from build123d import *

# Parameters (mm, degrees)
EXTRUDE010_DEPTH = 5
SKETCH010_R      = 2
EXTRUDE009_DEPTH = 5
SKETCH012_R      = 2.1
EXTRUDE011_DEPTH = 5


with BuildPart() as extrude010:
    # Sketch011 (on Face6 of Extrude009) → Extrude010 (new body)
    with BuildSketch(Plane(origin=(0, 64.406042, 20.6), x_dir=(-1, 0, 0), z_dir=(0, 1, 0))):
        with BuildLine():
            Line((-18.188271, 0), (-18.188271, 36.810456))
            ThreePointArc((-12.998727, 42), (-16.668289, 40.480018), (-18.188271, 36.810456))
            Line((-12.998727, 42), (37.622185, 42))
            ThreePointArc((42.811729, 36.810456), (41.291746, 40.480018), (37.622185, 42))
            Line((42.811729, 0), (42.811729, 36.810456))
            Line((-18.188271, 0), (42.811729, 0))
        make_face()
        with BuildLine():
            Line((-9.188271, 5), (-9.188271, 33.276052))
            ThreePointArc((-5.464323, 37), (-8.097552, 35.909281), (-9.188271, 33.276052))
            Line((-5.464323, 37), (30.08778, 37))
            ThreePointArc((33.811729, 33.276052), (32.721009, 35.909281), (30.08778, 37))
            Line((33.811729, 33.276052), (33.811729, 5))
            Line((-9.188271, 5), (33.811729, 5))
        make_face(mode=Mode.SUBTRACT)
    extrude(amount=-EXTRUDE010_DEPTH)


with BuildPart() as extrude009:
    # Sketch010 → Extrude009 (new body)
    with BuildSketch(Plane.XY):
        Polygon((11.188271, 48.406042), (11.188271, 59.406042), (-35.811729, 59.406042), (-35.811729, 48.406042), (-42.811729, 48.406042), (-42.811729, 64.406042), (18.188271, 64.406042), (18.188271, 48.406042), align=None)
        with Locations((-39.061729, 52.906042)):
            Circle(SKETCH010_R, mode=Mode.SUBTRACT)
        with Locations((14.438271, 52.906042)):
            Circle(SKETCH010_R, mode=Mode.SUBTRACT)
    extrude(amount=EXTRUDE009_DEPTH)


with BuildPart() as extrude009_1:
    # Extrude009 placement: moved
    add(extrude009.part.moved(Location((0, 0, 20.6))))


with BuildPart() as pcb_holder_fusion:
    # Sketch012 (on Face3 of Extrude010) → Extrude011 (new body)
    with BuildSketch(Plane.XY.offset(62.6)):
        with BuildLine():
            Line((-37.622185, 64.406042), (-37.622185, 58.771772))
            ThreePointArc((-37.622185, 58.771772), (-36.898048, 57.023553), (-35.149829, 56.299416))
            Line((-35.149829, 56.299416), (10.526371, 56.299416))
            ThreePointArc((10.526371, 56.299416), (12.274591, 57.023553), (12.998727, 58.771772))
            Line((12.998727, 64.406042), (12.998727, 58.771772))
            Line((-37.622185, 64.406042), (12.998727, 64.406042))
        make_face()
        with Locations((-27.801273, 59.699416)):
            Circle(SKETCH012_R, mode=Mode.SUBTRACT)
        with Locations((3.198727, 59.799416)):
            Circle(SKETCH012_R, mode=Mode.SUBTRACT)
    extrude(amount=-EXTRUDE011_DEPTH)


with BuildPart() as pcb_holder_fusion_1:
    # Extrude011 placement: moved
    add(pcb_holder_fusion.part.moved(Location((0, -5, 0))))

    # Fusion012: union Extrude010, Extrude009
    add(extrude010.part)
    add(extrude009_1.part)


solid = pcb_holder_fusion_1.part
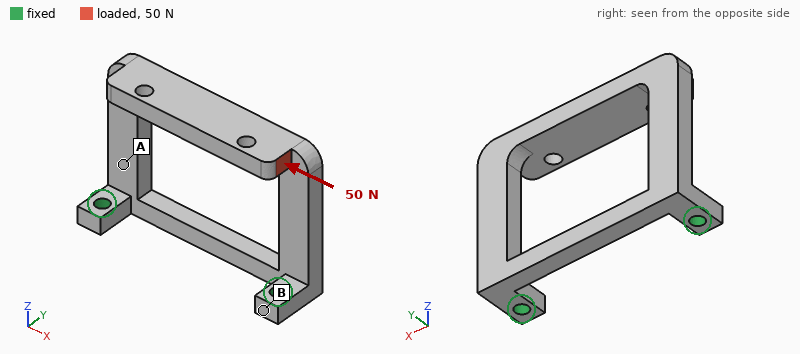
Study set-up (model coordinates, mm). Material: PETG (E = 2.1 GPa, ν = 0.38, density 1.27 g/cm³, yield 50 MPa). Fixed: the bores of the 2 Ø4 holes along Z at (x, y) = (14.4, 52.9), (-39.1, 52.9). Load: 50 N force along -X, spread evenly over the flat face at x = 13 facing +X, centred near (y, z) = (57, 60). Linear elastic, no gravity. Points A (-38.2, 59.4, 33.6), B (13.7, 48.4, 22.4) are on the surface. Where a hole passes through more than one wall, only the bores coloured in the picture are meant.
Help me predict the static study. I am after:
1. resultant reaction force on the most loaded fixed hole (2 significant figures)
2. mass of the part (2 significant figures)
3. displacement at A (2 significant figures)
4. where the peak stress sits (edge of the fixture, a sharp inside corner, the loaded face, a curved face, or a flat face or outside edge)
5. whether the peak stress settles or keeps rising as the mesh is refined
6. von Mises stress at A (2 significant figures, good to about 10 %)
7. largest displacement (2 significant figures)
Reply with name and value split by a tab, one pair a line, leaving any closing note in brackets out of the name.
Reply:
resultant reaction force on the most loaded fixed hole	35 N
mass of the part	11 g
displacement at A	0.19 mm
where the peak stress sits	edge of the fixture
whether the peak stress settles or keeps rising as the mesh is refined	keeps rising
von Mises stress at A	3.1 MPa
largest displacement	0.81 mm
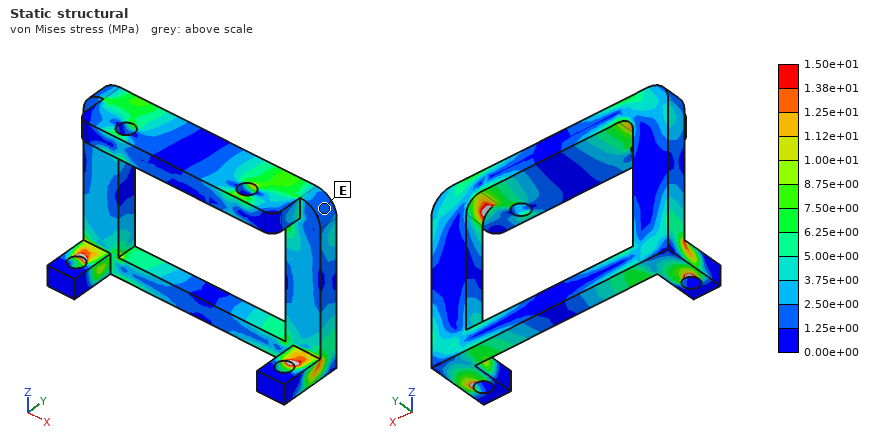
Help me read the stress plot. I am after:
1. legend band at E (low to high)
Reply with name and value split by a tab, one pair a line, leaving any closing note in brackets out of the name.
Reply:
legend band at E	1.25e+00 to 2.50e+00 MPa
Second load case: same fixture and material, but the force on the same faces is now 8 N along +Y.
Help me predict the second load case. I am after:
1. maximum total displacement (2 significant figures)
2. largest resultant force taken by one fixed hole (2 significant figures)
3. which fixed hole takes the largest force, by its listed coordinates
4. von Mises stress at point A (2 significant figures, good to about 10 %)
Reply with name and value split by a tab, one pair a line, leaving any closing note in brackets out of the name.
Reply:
maximum total displacement	0.80 mm
largest resultant force taken by one fixed hole	7.2 N
which fixed hole takes the largest force, by its listed coordinates	(14.4, 52.9)
von Mises stress at point A	2.2 MPa
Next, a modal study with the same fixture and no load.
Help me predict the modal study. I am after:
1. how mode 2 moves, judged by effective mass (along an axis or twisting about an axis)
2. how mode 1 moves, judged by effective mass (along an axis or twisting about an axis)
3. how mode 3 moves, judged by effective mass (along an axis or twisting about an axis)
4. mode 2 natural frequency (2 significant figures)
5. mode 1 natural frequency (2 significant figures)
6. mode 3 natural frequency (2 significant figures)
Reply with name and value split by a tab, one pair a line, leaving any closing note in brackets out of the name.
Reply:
how mode 2 moves, judged by effective mass	along X
how mode 1 moves, judged by effective mass	along Y
how mode 3 moves, judged by effective mass	along X
mode 2 natural frequency	560 Hz
mode 1 natural frequency	260 Hz
mode 3 natural frequency	700 Hz
